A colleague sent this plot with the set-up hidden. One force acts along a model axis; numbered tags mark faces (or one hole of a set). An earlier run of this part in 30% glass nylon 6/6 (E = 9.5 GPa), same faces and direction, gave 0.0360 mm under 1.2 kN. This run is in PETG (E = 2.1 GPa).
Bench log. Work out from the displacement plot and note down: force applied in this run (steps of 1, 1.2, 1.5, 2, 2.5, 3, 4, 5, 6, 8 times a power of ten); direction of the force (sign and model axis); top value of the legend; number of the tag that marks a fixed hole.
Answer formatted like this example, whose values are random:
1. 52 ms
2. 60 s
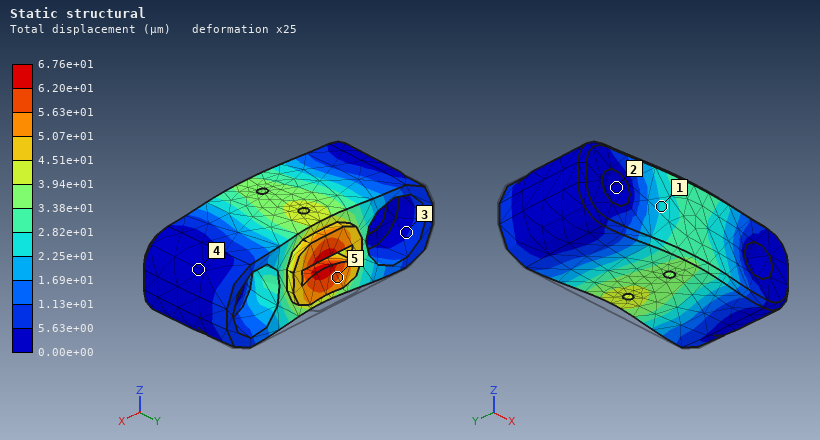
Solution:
1. 500 N
2. -Y
3. 6.76e+01 µm
4. 2
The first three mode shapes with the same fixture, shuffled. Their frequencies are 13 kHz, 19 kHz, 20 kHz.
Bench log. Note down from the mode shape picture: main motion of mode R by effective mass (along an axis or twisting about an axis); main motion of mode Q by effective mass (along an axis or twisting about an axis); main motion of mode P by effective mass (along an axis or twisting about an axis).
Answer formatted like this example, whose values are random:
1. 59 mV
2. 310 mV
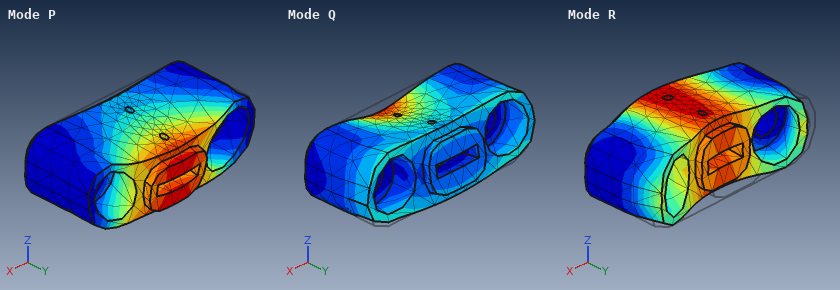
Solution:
1. along Y
2. along Z
3. along Z
